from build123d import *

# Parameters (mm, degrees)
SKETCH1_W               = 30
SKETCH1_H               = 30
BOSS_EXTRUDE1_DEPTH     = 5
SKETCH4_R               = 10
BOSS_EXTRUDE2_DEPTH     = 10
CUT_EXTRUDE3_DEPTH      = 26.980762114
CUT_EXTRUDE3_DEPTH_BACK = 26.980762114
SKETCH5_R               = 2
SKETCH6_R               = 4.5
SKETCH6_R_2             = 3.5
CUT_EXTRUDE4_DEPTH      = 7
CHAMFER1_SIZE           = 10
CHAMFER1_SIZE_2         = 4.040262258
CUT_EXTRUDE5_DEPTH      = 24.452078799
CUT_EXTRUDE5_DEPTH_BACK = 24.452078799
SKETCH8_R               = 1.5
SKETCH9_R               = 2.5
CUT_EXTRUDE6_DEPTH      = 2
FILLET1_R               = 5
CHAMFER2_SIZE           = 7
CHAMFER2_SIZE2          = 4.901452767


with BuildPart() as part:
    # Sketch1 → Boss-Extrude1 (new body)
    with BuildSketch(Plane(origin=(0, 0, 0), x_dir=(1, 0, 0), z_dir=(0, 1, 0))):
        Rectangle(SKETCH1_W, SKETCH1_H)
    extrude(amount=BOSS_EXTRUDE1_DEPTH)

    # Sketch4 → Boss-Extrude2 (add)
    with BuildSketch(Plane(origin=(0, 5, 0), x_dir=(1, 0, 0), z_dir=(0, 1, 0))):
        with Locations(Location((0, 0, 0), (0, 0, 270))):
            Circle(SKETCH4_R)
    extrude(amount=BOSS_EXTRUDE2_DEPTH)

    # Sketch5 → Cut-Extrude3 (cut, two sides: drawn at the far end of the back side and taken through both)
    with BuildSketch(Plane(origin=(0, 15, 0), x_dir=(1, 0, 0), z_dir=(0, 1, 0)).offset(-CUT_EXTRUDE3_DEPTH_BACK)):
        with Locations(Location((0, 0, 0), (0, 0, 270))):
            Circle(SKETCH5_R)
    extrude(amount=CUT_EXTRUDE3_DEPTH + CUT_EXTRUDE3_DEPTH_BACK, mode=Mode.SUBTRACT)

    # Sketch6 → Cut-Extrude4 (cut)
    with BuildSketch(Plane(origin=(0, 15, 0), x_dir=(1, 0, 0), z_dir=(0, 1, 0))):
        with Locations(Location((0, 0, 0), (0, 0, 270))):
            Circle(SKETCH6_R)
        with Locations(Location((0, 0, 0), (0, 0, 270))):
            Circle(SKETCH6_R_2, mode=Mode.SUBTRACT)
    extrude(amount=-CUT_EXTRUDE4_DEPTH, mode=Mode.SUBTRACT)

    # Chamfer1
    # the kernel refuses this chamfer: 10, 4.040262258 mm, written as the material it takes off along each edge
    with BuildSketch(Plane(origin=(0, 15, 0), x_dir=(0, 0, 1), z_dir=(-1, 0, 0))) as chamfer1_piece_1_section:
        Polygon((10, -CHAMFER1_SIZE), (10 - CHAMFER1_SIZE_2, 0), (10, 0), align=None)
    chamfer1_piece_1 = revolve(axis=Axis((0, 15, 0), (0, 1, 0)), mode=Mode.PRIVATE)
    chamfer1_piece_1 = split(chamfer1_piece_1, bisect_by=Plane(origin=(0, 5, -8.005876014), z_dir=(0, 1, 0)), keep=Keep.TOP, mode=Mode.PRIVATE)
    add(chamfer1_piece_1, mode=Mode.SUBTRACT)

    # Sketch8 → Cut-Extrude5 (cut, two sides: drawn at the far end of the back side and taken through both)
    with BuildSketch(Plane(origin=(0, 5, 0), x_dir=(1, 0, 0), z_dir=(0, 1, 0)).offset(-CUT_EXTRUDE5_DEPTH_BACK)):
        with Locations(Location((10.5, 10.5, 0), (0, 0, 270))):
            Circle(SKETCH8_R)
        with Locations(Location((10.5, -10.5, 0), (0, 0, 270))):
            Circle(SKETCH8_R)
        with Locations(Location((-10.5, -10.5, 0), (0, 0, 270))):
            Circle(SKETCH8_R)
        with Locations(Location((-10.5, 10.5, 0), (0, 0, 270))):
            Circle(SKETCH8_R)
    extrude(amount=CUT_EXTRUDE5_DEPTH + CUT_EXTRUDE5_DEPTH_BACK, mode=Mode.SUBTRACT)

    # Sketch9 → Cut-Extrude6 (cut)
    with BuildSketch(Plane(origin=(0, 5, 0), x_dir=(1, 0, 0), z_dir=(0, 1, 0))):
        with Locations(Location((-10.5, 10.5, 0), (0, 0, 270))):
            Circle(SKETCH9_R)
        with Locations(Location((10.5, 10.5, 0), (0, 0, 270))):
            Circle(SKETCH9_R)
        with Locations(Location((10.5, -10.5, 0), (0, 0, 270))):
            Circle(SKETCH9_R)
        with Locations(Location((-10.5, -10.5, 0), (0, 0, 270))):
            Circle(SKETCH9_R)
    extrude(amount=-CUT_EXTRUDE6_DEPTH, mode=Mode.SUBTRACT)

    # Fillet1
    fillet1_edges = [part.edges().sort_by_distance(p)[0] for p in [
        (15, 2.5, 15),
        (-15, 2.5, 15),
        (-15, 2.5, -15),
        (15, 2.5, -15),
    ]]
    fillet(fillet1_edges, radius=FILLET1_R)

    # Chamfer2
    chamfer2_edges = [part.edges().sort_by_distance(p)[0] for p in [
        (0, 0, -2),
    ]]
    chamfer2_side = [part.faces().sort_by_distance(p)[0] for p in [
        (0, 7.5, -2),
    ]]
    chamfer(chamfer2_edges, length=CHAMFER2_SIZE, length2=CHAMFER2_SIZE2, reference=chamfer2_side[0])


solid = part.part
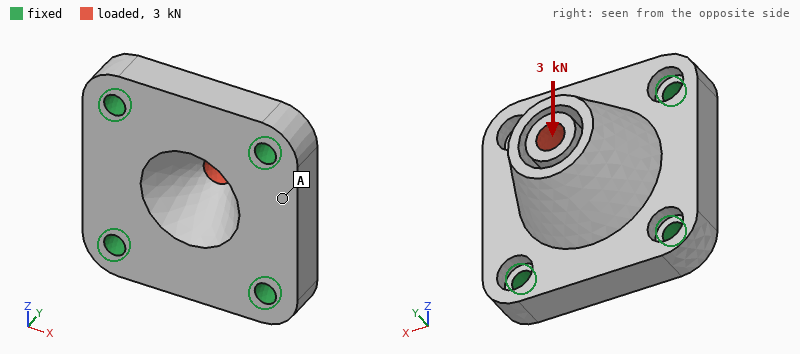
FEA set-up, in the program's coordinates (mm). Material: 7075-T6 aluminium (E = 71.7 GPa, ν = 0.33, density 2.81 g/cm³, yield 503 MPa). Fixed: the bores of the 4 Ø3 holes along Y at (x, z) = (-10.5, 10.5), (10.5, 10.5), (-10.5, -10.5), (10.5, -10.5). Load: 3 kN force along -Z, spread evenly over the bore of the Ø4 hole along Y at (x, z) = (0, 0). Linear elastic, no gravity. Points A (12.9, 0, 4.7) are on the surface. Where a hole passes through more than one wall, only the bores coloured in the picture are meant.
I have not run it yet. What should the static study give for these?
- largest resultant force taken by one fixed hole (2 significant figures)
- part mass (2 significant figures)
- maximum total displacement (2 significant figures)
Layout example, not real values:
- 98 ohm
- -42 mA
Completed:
- 1.2 kN
- 15 g
- 74 µm
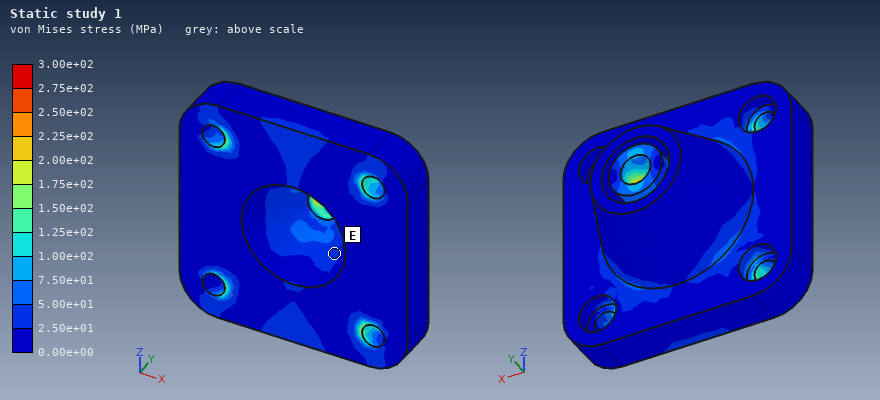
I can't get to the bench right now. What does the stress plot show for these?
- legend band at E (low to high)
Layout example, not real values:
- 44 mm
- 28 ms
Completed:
- 2.50e+01 to 5.00e+01 MPa
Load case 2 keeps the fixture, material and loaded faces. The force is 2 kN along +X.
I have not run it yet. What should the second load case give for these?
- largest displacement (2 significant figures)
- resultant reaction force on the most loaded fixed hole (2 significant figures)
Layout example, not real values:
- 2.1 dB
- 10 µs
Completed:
- 49 µm
- 770 N
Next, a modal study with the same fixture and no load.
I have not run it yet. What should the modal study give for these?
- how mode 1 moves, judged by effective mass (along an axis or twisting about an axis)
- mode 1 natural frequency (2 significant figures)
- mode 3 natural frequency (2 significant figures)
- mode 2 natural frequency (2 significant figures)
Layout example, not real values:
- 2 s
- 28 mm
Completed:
- along Y
- 29 kHz
- 33 kHz
- 33 kHz
